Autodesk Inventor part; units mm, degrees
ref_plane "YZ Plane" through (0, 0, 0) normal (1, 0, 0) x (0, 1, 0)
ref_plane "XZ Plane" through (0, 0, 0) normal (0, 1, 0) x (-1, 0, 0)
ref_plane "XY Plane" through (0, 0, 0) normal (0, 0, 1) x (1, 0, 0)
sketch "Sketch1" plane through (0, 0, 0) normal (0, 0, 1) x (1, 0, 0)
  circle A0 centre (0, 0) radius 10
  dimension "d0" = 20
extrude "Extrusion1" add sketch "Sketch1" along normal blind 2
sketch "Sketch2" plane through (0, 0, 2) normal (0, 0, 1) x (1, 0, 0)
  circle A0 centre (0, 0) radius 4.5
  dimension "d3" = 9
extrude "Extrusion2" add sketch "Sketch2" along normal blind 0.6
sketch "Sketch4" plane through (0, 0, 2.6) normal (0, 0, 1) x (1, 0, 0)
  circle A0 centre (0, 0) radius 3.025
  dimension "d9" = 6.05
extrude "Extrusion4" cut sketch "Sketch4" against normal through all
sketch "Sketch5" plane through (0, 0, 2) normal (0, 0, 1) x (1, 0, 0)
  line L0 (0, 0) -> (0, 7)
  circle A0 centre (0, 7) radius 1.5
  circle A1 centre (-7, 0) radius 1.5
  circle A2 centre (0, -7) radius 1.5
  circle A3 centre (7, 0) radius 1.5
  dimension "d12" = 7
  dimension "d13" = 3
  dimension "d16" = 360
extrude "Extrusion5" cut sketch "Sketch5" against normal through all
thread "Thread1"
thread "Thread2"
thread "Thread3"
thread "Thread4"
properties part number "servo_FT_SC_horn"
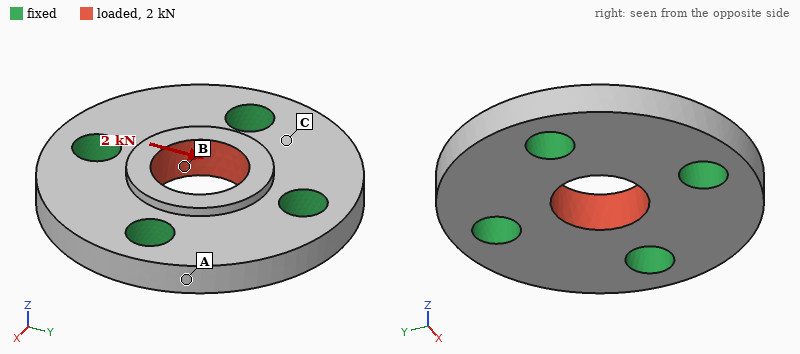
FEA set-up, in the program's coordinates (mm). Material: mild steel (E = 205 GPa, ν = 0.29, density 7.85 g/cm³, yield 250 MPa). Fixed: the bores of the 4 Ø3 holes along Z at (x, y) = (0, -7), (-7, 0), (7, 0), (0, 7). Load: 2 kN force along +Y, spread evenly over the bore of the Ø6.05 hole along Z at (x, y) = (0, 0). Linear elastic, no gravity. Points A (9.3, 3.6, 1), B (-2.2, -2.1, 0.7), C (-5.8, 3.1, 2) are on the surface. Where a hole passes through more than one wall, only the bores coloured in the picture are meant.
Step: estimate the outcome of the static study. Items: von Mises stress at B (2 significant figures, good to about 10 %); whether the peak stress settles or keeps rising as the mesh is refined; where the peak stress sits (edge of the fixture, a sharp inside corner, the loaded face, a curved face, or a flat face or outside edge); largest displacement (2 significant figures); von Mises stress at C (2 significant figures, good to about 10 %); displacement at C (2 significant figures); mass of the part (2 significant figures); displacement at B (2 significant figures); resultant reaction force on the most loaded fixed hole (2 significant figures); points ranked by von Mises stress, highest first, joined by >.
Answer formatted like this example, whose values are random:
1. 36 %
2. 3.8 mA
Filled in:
1. 62 MPa
2. keeps rising
3. a sharp inside corner
4. 1.4 µm
5. 23 MPa
6. 0.40 µm
7. 4.2 g
8. 1.1 µm
9. 620 N
10. B > C > A
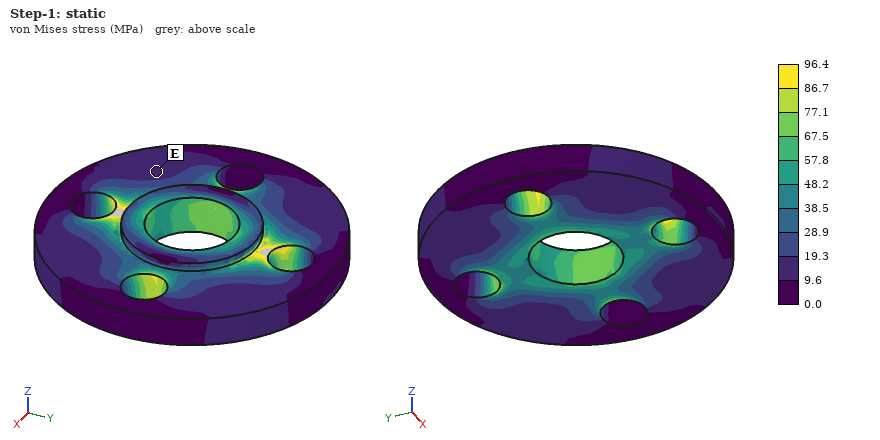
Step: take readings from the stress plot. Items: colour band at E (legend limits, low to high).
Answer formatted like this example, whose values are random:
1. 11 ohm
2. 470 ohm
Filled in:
1. 9.6 to 19.3 MPa
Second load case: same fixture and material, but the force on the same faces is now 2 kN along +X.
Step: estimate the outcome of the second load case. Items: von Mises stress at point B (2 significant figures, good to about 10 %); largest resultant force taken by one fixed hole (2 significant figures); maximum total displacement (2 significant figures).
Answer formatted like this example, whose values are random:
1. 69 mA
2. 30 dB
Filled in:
1. 61 MPa
2. 620 N
3. 1.4 µm
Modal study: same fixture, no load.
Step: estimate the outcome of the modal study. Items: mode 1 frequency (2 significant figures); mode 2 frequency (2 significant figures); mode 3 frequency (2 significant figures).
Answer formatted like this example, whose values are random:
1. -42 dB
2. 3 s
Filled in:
1. 77 kHz
2. 77 kHz
3. 77 kHz
